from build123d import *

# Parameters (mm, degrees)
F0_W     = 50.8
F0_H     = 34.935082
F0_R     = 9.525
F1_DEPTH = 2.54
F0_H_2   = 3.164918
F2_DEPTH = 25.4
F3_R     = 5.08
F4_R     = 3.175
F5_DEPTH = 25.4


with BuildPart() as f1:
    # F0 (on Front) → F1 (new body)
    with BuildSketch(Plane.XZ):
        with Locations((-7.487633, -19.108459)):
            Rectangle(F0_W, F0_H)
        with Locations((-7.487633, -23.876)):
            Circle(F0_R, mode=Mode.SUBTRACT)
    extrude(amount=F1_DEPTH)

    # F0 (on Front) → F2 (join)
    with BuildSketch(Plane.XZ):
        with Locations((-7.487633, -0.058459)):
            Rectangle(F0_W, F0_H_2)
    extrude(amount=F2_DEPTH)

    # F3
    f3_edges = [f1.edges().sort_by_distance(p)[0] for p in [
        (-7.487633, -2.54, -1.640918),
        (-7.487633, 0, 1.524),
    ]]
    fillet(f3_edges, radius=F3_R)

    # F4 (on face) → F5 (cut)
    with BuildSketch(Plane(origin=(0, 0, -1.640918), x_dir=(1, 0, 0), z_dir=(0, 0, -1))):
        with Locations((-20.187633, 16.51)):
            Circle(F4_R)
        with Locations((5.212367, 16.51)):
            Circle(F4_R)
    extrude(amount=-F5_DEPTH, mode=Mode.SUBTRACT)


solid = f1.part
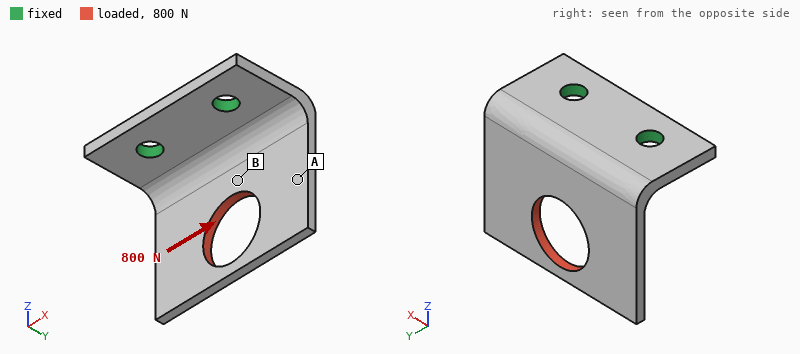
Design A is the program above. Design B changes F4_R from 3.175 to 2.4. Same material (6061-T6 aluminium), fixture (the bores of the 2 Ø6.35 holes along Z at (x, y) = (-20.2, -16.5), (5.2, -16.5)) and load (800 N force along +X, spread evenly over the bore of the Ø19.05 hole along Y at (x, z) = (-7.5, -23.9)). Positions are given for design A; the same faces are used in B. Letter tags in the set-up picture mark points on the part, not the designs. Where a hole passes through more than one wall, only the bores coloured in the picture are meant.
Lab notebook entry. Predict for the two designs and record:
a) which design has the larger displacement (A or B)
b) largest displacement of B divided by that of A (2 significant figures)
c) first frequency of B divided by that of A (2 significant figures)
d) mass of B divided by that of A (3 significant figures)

B
1.1
0.97
1.01
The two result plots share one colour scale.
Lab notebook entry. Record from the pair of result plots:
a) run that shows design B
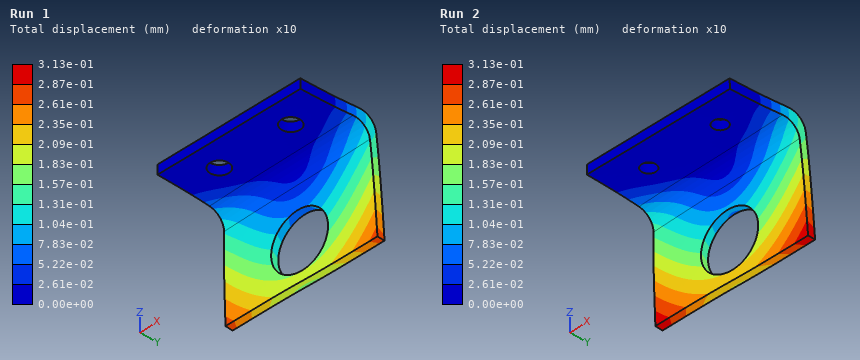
Run 2
